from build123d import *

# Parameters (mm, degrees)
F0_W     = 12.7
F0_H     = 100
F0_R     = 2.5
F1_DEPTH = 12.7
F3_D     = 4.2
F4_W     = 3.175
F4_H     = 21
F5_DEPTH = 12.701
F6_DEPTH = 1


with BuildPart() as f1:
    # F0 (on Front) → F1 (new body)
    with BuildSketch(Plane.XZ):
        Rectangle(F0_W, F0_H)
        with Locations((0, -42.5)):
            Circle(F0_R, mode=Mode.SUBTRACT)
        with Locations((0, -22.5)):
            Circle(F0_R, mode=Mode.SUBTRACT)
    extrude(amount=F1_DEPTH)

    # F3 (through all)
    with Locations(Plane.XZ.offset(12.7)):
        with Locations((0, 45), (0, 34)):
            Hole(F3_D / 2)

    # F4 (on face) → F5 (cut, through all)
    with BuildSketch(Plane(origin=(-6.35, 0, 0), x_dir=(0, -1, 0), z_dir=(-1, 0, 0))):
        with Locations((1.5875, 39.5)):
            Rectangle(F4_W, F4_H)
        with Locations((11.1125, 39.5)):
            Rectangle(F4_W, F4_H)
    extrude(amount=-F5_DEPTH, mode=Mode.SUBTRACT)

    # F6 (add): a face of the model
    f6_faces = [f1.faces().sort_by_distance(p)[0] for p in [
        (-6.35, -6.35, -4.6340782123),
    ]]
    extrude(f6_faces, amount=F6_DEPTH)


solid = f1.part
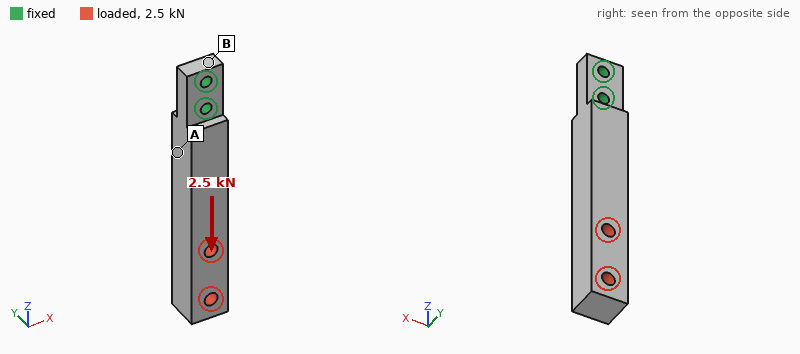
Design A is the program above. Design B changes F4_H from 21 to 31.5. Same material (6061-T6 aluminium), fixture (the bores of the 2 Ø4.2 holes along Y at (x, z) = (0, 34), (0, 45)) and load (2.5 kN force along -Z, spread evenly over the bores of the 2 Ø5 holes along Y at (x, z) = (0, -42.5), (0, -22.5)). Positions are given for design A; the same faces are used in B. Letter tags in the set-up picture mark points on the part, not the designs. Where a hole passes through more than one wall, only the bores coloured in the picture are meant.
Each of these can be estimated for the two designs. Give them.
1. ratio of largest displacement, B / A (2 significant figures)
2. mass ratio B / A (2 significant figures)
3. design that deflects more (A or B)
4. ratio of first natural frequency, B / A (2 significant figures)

1.1
0.97
B
0.84
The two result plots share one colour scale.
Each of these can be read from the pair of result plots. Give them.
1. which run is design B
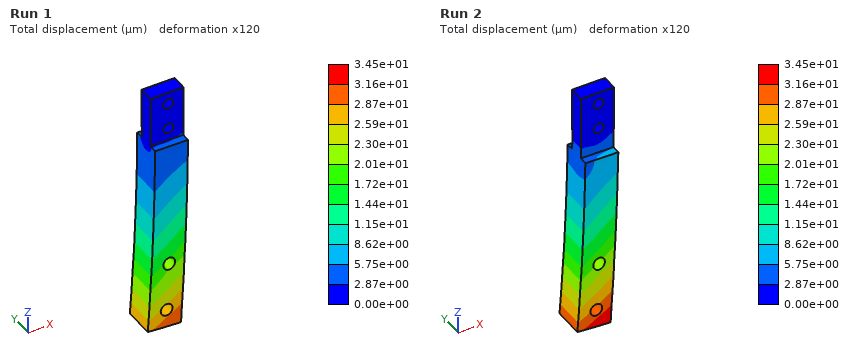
Run 2
